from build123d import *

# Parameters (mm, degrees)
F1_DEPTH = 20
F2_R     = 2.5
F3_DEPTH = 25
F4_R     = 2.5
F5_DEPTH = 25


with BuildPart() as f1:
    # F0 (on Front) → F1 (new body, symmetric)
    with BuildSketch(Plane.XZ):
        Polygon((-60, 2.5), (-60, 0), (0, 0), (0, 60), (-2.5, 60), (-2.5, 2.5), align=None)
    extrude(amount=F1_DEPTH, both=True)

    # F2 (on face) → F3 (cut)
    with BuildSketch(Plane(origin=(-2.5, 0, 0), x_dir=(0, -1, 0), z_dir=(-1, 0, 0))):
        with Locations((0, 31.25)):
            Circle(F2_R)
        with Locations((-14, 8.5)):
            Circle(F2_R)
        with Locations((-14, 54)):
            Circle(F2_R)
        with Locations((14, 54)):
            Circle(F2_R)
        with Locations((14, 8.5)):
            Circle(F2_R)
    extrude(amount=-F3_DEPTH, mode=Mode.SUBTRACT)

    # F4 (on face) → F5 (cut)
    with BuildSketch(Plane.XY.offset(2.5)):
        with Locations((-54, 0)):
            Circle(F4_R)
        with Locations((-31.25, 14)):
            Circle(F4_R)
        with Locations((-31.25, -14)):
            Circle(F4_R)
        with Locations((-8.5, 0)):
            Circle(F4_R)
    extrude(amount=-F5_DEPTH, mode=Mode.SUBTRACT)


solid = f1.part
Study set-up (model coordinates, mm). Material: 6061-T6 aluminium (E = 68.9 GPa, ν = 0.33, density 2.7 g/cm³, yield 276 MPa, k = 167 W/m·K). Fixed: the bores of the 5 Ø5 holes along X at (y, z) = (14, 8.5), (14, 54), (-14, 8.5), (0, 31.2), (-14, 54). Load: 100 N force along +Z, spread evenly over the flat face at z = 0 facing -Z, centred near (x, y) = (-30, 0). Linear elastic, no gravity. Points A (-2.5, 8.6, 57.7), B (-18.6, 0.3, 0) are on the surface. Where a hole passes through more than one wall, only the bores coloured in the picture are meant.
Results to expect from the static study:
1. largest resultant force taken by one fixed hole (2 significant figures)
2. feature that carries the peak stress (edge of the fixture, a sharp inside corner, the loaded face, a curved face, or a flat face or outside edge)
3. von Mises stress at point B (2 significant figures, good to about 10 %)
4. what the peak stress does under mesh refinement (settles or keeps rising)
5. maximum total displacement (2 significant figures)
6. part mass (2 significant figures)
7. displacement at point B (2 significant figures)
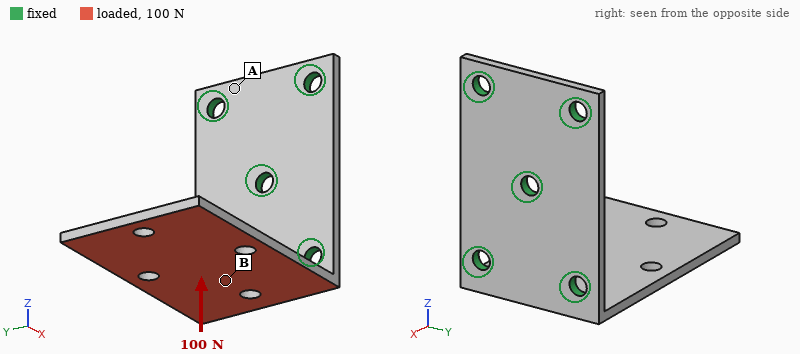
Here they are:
40 N
edge of the fixture
28 MPa
keeps rising
0.94 mm
31 g
0.18 mm
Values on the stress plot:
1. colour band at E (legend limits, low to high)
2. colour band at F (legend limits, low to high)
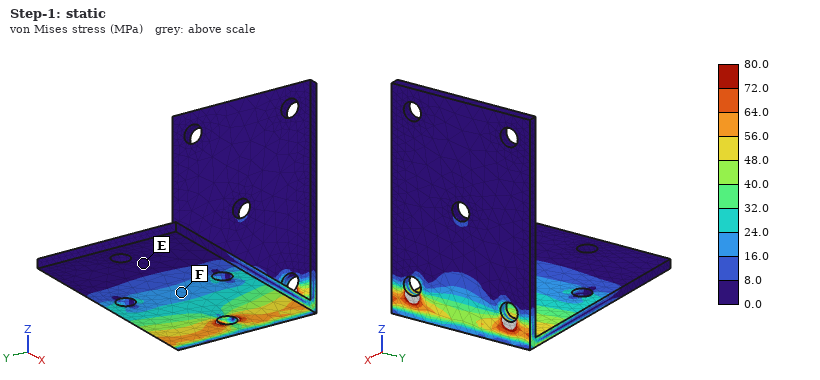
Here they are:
0.0 to 8.0 MPa
16.0 to 24.0 MPa
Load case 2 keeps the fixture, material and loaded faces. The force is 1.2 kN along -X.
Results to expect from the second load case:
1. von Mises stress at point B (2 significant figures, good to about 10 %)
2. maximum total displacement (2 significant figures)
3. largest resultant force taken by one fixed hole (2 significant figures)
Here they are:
26 MPa
0.99 mm
620 N
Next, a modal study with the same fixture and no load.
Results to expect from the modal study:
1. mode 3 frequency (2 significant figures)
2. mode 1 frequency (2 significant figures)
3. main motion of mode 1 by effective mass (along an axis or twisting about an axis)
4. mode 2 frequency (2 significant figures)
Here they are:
3200 Hz
520 Hz
along Z
1800 Hz
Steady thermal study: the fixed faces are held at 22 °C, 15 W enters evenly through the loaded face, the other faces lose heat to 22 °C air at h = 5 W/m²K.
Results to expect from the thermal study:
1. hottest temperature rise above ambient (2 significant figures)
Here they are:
33 K
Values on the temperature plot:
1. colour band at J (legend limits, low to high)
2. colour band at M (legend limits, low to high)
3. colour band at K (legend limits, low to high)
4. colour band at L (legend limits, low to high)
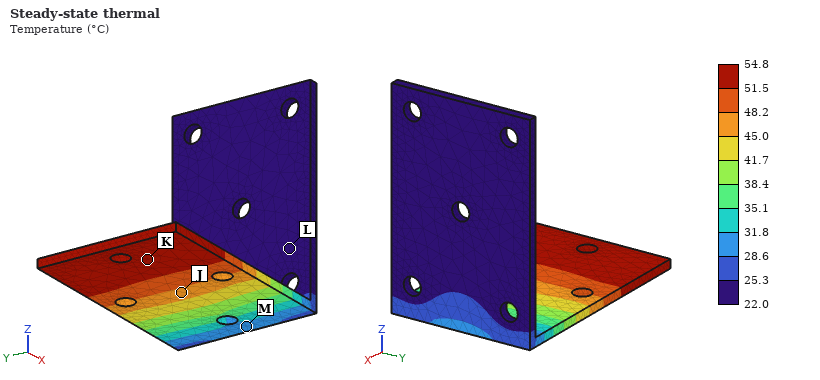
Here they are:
45.0 to 48.2 °C
28.6 to 31.8 °C
51.5 to 54.8 °C
22.0 to 25.3 °C
